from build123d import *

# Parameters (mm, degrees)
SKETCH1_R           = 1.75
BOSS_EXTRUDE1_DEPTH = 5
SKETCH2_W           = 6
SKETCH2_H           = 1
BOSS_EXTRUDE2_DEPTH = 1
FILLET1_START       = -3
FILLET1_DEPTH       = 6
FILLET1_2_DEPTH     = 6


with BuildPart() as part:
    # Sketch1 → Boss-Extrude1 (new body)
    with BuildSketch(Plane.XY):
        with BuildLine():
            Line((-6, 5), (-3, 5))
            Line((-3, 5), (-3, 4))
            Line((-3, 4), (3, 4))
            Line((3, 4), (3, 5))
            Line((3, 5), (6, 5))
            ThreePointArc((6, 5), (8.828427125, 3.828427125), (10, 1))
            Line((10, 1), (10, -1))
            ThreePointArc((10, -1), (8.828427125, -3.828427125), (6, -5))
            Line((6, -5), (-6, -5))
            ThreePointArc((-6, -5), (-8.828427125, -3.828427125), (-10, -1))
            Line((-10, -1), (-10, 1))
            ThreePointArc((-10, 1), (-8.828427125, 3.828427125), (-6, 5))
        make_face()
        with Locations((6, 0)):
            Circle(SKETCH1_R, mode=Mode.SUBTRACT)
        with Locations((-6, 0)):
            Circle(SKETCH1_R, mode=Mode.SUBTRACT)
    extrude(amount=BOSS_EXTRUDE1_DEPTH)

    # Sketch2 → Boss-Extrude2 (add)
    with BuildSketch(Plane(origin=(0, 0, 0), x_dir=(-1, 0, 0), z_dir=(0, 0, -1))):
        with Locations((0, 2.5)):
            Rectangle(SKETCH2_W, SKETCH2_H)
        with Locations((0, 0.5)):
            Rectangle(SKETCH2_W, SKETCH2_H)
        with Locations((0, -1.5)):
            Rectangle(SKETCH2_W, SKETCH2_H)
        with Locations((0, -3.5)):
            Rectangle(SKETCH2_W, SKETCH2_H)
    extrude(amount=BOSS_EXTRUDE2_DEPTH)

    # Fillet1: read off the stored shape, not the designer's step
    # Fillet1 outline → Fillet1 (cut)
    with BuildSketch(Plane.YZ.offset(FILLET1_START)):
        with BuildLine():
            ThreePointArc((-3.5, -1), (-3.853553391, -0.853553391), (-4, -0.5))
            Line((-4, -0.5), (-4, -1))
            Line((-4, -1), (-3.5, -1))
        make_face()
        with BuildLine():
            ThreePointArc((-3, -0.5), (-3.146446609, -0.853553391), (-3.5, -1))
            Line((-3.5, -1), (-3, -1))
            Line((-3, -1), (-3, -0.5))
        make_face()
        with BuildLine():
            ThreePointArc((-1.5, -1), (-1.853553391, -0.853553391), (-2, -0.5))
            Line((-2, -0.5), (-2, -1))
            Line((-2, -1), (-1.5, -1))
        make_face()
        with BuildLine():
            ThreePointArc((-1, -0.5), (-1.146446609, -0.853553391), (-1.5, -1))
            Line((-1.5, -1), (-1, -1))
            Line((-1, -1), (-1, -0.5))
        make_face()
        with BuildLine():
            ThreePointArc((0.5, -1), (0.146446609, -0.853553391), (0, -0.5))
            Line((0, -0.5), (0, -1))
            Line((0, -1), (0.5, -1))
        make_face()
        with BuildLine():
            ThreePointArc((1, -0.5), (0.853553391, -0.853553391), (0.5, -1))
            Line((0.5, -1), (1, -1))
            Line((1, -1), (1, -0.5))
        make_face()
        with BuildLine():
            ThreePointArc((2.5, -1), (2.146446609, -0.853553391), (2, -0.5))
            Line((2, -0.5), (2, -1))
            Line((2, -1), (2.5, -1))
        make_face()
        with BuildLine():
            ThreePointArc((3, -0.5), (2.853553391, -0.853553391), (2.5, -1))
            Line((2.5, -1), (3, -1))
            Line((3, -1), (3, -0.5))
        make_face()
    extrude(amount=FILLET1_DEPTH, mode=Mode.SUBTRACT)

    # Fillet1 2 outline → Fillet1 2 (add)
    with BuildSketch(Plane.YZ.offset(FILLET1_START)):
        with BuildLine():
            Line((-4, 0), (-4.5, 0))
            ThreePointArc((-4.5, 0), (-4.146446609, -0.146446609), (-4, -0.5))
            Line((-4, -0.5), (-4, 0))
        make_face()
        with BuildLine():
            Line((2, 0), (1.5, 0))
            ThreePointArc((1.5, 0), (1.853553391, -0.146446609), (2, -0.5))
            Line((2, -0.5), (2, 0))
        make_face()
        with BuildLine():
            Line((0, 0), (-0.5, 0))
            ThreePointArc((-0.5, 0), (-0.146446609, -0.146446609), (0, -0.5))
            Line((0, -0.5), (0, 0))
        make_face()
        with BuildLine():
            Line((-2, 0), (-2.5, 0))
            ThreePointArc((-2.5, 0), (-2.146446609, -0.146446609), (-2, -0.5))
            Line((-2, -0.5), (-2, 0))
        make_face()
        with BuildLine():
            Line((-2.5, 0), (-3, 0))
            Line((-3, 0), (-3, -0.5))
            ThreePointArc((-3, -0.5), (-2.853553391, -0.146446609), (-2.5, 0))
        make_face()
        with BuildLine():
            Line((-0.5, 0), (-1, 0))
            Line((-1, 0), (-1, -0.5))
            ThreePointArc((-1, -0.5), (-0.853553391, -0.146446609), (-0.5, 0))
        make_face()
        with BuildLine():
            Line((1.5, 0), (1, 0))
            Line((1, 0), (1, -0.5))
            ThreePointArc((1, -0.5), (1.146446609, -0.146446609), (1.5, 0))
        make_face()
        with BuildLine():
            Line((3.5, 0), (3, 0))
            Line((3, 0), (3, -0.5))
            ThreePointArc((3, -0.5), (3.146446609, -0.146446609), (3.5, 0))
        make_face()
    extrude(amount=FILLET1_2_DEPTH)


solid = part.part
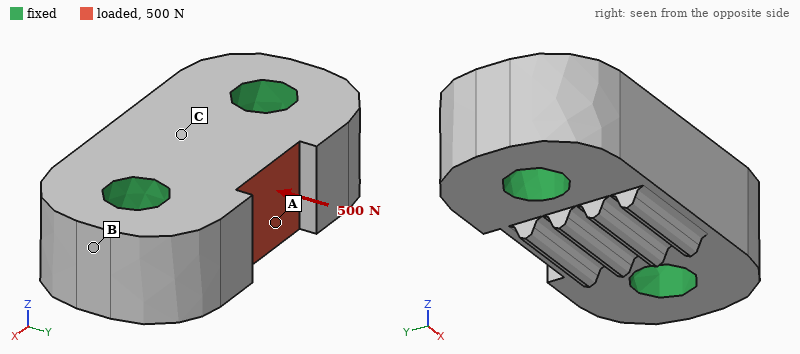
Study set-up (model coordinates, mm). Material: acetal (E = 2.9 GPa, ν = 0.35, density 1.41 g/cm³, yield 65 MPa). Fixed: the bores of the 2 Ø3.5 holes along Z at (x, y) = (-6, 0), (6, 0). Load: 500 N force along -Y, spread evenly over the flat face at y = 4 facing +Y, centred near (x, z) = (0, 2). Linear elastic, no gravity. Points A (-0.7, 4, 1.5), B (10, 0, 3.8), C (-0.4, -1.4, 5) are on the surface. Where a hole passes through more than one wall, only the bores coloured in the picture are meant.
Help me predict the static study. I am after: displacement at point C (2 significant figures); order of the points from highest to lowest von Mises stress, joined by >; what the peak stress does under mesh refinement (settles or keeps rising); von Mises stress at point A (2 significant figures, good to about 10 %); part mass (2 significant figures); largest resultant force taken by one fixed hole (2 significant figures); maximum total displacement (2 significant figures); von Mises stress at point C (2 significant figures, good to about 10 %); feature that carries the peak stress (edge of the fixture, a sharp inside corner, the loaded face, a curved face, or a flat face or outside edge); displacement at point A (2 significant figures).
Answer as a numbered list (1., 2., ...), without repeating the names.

1. 20 µm
2. A > C > B
3. keeps rising
4. 15 MPa
5. 1.2 g
6. 260 N
7. 41 µm
8. 6.0 MPa
9. edge of the fixture
10. 36 µm
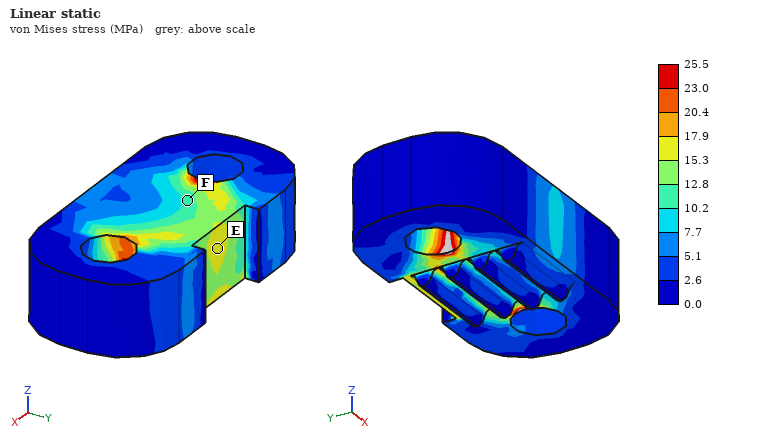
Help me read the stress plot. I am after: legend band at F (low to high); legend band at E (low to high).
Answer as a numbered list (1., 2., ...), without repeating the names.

1. 10.2 to 12.8 MPa
2. 15.3 to 17.9 MPa
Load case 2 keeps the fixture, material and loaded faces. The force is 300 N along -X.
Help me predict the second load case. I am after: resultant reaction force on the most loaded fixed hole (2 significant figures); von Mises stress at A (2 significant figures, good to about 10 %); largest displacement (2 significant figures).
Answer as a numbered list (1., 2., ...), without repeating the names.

1. 170 N
2. 18 MPa
3. 21 µm
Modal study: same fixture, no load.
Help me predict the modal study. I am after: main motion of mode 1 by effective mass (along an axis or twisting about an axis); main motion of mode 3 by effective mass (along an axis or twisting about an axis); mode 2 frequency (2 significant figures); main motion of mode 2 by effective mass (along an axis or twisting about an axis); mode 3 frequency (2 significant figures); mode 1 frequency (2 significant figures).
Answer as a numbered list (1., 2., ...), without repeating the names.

1. along Z
2. along Y
3. 33 kHz
4. along Z
5. 35 kHz
6. 29 kHz
